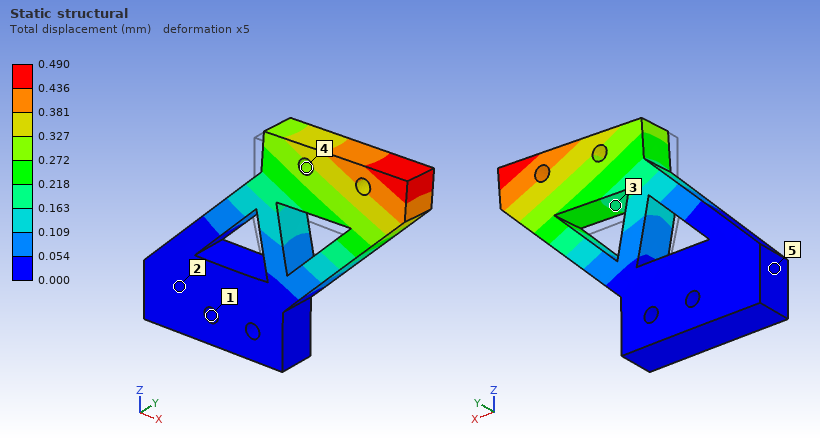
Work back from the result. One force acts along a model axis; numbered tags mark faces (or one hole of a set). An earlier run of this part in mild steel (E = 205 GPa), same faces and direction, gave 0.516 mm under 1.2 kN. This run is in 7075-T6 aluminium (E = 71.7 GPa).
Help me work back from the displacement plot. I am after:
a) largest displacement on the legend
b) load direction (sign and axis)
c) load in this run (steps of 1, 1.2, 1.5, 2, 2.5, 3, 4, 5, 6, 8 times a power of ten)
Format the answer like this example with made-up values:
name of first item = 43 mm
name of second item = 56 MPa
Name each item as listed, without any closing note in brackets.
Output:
largest displacement on the legend = 0.490 mm
load direction = +Y
load in this run = 400 N
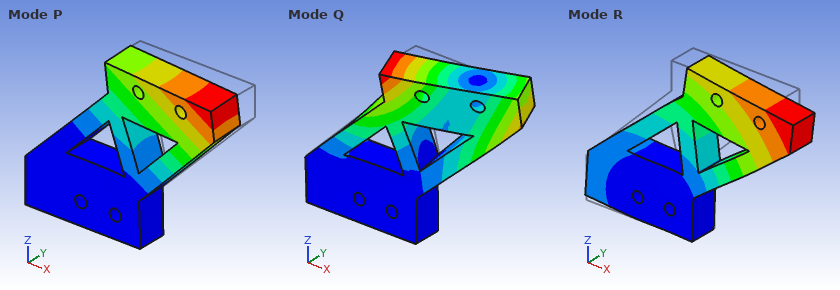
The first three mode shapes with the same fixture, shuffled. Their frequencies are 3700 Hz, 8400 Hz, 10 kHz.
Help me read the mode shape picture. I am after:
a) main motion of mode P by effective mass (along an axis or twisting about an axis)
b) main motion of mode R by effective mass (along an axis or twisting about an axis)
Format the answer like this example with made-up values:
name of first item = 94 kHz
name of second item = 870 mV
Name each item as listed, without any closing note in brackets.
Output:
main motion of mode P by effective mass = along Y
main motion of mode R by effective mass = along X
